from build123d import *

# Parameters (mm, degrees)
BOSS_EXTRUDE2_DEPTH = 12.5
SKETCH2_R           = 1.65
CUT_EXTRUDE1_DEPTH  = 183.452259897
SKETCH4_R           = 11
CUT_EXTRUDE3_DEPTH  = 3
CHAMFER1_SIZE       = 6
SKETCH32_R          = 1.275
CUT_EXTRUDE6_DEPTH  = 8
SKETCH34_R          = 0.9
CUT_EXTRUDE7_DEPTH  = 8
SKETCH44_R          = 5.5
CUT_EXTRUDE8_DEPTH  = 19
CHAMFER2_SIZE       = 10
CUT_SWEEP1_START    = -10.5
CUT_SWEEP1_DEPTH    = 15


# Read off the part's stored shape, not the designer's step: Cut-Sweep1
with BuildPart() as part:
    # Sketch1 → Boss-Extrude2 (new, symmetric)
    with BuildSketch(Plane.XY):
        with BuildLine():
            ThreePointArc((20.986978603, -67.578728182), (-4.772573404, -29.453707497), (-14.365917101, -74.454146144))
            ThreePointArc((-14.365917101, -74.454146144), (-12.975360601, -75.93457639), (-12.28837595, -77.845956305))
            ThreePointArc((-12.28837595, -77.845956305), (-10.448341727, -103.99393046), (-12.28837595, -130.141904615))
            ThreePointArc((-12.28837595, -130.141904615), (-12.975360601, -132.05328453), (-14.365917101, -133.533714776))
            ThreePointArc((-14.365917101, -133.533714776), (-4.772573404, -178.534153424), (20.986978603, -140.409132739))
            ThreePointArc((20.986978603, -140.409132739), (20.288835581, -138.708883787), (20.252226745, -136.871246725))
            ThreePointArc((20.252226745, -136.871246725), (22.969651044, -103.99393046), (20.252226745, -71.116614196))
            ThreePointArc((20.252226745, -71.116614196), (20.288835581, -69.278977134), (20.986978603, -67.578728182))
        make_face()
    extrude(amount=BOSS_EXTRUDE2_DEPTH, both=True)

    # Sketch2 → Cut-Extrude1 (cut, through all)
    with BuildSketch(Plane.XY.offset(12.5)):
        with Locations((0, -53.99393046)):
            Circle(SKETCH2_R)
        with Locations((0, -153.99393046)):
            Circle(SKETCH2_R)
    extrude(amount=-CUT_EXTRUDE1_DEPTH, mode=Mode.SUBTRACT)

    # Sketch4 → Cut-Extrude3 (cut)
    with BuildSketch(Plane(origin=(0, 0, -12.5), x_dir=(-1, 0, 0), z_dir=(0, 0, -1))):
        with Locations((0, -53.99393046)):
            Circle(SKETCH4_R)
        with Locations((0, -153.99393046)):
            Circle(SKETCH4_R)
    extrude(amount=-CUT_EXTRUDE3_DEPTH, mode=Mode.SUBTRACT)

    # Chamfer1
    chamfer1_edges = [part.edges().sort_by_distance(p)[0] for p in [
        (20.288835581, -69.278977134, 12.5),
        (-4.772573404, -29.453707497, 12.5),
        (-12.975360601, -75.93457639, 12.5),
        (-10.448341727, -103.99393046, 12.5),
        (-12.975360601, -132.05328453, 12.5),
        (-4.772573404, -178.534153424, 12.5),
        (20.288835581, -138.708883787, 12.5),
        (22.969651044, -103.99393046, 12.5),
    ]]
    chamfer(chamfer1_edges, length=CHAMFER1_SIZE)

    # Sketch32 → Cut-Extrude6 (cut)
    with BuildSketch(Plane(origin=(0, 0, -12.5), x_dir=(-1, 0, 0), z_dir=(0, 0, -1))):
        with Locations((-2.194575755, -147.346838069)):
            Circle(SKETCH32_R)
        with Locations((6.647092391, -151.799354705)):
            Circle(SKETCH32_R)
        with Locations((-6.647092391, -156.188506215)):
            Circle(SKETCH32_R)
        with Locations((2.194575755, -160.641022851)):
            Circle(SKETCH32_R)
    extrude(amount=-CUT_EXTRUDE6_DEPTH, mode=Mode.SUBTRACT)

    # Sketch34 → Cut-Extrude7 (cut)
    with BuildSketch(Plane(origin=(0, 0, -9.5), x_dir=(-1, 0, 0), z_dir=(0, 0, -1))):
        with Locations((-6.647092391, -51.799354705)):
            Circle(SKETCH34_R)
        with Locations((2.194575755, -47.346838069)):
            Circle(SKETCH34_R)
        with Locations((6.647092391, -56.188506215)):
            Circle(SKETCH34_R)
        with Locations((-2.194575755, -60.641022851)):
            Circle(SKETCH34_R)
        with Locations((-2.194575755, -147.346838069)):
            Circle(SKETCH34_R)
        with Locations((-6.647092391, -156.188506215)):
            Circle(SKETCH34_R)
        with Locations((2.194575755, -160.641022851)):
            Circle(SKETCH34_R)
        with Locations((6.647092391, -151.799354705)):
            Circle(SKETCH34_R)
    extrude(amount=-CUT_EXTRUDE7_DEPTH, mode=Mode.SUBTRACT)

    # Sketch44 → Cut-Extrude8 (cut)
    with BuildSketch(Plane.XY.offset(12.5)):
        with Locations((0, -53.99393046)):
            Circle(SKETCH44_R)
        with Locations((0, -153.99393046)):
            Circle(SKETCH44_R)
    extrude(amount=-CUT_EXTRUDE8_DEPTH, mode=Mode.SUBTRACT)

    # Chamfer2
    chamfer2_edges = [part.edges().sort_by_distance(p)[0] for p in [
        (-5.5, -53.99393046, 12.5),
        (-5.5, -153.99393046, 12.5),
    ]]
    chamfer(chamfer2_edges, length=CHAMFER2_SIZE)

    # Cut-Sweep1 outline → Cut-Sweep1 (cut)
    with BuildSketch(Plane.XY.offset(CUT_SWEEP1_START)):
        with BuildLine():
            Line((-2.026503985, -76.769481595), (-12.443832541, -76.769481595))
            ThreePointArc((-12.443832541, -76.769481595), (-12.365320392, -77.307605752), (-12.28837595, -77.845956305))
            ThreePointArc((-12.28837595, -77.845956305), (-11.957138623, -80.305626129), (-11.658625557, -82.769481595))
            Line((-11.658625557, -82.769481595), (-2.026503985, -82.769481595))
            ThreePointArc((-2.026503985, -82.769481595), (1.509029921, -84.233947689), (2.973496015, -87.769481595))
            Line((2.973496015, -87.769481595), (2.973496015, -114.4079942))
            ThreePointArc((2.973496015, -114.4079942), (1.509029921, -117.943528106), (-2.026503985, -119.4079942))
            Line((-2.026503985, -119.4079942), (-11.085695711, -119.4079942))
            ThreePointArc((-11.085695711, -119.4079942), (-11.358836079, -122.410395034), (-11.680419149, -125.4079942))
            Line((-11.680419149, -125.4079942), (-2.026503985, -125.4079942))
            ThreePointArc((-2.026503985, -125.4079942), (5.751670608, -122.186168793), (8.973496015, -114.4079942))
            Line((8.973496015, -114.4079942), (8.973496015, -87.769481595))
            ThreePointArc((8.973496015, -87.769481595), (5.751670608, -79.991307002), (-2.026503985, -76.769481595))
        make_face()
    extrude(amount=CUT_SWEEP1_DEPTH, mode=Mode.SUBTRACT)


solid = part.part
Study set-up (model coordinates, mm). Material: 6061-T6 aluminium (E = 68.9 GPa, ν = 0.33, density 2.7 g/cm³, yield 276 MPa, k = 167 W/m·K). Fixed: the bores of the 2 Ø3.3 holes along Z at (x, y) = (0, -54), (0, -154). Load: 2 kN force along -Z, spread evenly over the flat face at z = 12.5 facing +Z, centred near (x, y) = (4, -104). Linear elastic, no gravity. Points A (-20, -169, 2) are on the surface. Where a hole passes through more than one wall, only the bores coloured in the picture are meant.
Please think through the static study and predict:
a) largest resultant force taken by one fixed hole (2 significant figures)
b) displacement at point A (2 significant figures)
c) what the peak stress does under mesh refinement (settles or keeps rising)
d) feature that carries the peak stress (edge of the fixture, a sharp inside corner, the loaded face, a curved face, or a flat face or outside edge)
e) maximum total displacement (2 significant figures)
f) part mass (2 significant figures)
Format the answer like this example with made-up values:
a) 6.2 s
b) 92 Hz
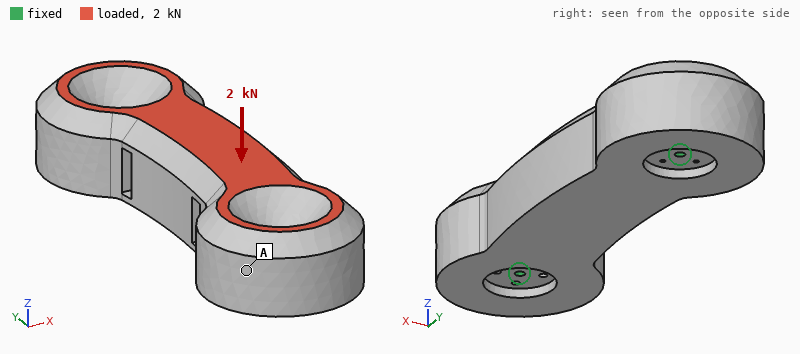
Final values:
a) 1.1 kN
b) 43 µm
c) keeps rising
d) edge of the fixture
e) 70 µm
f) 320 g
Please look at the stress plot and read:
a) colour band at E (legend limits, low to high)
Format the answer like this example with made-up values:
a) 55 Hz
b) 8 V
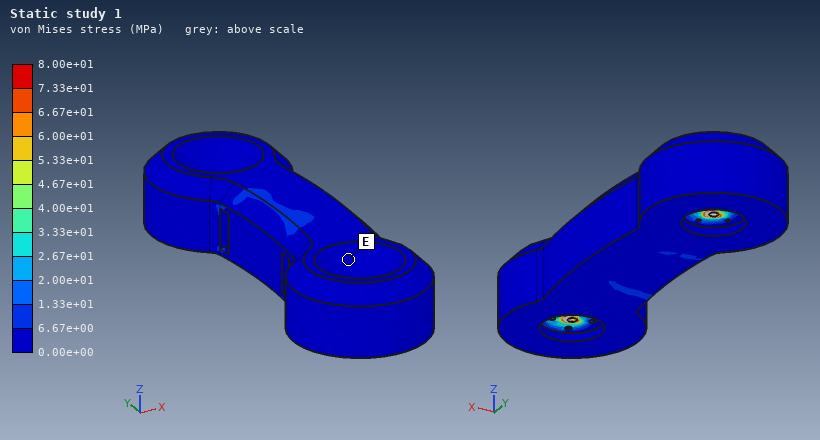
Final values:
a) 0.00e+00 to 6.67e+00 MPa
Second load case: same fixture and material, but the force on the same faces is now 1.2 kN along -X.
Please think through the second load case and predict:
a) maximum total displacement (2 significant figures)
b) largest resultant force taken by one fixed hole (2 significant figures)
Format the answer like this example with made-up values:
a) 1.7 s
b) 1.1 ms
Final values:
a) 0.21 mm
b) 630 N
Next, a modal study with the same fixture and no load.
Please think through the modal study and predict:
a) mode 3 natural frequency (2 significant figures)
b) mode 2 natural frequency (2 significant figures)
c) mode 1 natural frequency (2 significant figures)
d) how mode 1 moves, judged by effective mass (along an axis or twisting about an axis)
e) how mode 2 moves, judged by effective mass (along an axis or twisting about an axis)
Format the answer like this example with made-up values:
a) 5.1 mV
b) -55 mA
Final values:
a) 5200 Hz
b) 4300 Hz
c) 1000 Hz
d) along X
e) along Z
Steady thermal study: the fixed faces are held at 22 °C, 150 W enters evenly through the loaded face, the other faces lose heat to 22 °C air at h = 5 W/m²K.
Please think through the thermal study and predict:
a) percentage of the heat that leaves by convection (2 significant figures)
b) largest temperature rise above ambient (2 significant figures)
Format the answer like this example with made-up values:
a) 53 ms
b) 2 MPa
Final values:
a) 3.2 %
b) 58 K
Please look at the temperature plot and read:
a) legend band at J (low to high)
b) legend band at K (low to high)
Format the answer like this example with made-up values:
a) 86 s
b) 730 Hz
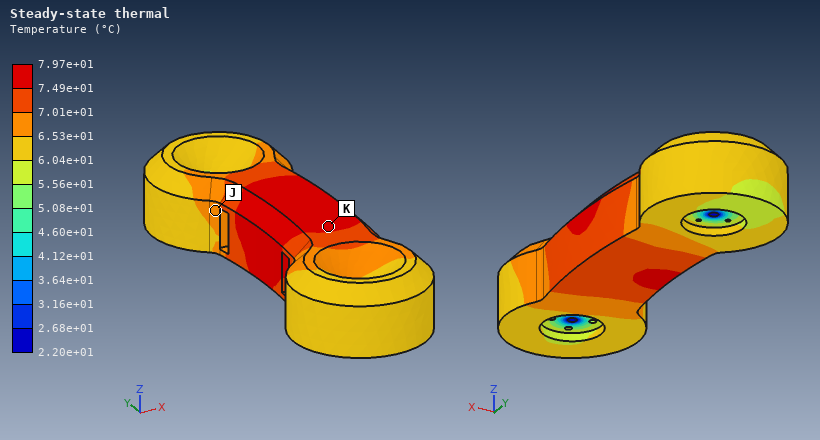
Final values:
a) 6.53e+01 to 7.01e+01 °C
b) 7.49e+01 to 7.97e+01 °C
